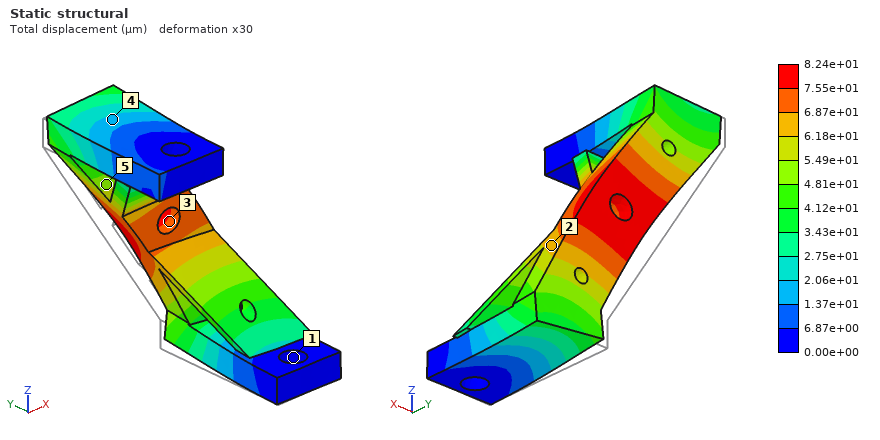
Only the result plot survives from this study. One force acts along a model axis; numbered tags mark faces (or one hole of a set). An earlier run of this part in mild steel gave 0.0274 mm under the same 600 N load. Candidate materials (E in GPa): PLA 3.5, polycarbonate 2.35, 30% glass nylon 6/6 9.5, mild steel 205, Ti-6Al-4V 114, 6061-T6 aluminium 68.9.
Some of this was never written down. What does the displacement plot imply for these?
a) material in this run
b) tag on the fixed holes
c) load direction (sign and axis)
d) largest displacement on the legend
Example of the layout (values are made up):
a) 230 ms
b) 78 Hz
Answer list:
a) 6061-T6 aluminium
b) 1
c) +X
d) 8.24e+01 µm
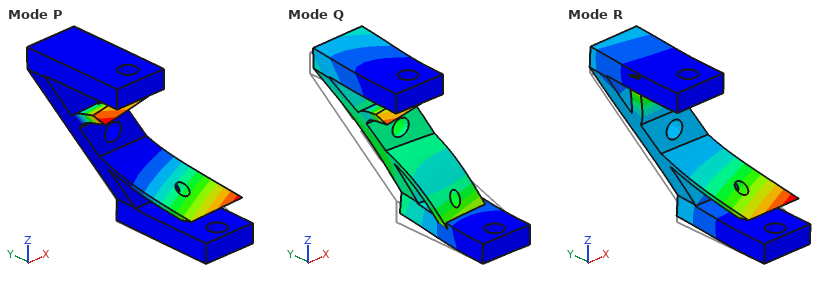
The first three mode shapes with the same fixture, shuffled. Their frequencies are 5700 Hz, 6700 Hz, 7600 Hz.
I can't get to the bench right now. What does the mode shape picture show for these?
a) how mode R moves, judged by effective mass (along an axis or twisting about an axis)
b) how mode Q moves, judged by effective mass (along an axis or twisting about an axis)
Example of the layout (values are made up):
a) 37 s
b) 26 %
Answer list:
a) along Z
b) along X
